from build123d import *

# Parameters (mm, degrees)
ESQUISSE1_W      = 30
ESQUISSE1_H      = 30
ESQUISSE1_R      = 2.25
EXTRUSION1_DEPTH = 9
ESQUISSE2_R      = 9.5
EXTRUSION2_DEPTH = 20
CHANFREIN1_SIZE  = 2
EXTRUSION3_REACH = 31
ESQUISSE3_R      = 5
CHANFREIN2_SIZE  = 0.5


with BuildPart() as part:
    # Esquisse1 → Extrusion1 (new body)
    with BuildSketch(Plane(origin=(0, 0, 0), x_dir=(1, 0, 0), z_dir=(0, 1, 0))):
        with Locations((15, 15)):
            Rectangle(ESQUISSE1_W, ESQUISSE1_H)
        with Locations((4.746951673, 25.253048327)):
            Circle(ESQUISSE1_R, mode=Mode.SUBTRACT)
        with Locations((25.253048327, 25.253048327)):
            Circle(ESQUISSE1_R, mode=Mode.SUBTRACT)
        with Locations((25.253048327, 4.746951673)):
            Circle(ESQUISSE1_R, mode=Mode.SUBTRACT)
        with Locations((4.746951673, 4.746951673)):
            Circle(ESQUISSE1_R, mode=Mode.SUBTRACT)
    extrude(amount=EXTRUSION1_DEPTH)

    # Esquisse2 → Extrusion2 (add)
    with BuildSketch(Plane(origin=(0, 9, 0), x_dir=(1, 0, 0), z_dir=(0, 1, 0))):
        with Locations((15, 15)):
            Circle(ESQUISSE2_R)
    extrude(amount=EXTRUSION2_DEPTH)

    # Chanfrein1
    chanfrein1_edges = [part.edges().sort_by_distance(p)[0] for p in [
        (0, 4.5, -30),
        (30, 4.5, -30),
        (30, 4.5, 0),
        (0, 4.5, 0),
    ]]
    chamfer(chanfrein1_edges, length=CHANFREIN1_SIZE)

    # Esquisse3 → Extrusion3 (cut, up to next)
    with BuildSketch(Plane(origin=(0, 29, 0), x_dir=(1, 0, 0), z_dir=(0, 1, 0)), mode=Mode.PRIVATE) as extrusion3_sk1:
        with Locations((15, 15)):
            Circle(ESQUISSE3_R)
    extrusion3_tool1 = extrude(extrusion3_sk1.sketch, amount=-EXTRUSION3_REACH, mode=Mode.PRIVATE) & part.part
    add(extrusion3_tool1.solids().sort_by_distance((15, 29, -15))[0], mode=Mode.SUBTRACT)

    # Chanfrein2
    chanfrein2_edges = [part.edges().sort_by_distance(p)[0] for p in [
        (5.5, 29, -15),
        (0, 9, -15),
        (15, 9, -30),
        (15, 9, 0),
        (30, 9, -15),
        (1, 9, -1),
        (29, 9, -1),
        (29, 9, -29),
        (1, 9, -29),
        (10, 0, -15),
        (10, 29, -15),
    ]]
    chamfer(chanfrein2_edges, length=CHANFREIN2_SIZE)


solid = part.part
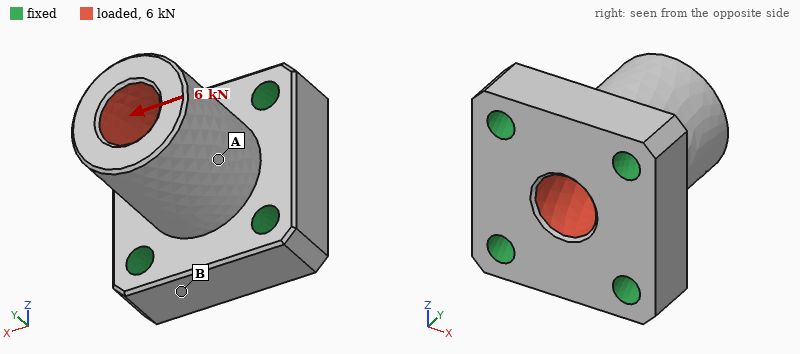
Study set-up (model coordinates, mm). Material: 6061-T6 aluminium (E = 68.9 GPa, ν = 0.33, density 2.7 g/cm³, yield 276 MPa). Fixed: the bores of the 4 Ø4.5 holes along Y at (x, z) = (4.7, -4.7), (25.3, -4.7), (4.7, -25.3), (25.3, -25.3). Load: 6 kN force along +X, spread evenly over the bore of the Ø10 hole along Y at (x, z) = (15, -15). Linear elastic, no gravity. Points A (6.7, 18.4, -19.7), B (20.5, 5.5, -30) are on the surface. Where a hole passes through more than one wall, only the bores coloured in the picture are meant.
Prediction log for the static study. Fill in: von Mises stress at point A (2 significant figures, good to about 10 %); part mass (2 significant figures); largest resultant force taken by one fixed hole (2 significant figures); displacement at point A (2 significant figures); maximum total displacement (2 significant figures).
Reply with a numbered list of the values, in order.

1. 19 MPa
2. 29 g
3. 2.2 kN
4. 23 µm
5. 39 µm
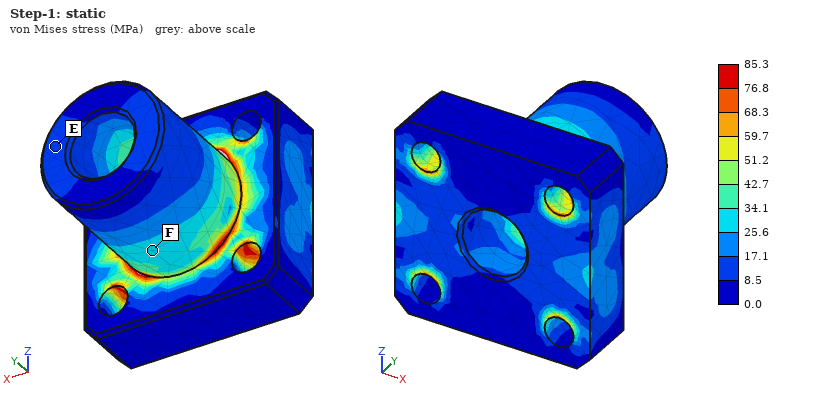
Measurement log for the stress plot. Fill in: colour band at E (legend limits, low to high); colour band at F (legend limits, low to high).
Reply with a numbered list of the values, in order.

1. 8.5 to 17.1 MPa
2. 25.6 to 34.1 MPa
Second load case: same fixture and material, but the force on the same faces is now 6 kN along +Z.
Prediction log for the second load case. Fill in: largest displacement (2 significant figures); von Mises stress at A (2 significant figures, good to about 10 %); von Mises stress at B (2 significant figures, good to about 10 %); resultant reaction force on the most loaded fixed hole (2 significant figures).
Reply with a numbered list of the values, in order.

1. 39 µm
2. 24 MPa
3. 23 MPa
4. 2.2 kN
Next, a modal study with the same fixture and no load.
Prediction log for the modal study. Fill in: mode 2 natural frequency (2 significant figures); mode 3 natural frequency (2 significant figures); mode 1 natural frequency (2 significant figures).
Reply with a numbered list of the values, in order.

1. 18 kHz
2. 34 kHz
3. 18 kHz
